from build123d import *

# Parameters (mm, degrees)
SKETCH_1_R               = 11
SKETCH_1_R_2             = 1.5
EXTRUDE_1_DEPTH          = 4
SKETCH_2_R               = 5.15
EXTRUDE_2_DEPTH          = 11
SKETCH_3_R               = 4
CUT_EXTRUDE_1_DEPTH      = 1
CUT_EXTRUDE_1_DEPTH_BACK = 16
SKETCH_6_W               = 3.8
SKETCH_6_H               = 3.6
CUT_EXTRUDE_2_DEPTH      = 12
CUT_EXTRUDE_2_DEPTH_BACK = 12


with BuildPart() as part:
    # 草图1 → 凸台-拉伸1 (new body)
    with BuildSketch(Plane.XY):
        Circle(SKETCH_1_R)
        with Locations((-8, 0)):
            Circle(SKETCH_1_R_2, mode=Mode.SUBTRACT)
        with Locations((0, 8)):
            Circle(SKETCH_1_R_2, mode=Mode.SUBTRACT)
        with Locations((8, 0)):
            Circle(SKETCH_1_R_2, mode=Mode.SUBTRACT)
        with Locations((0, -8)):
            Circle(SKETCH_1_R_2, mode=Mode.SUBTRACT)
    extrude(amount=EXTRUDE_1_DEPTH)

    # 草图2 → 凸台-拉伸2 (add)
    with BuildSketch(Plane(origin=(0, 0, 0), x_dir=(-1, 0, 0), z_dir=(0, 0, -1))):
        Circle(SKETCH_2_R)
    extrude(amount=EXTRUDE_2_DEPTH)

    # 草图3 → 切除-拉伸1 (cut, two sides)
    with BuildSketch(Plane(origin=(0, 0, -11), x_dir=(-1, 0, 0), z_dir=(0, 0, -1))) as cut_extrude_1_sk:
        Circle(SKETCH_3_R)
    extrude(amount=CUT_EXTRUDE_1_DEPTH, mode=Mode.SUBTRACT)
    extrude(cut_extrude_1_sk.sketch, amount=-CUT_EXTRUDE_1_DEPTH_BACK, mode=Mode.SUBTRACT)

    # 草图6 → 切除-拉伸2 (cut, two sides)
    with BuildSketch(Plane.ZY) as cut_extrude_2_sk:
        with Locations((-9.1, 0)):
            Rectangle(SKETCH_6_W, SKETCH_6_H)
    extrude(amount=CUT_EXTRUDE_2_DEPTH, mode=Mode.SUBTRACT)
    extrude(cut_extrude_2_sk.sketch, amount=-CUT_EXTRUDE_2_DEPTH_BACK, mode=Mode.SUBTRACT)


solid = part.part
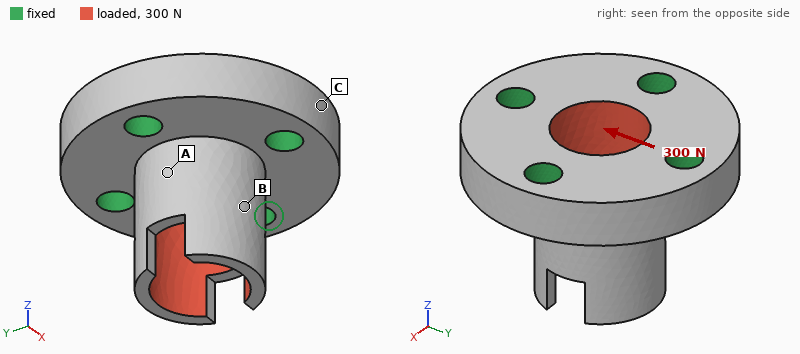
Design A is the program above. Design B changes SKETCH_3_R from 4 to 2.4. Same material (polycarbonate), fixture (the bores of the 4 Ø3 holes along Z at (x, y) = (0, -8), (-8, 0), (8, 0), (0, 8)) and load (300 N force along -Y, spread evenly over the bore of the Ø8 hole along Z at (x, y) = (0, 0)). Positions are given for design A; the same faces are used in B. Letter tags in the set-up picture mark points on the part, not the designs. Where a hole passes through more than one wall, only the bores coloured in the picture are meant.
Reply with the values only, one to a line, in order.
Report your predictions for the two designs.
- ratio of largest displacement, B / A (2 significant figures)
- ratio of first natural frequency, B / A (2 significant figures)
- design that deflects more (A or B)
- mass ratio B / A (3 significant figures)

0.49
1.1
A
1.28
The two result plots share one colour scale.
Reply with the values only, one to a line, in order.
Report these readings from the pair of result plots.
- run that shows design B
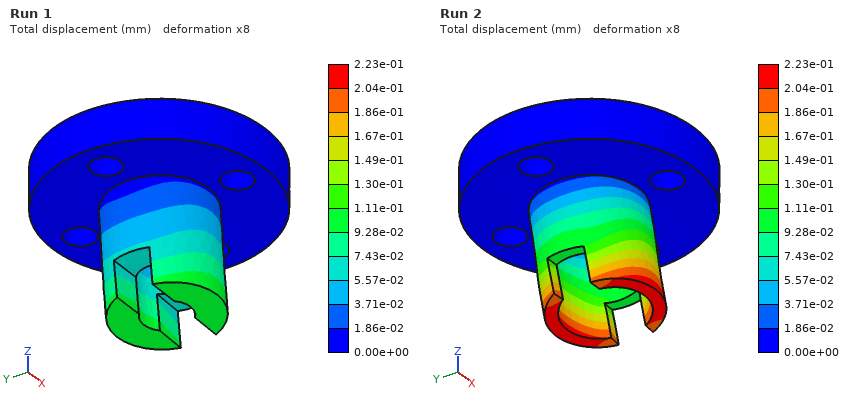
Run 1
